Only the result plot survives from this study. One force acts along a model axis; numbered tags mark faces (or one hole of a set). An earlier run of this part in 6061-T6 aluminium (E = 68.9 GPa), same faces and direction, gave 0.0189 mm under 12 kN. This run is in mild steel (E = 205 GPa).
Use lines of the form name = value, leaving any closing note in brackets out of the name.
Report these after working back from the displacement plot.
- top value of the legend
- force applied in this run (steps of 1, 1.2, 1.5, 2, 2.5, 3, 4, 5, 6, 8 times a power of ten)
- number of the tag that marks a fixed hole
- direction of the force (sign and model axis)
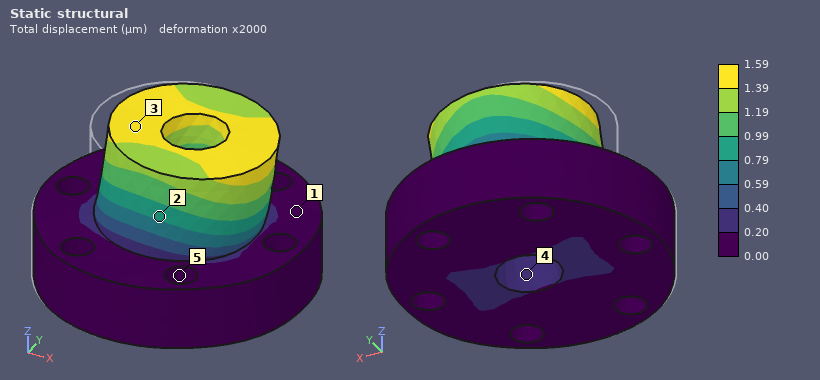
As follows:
top value of the legend = 1.59 µm
force applied in this run = 3 kN
number of the tag that marks a fixed hole = 5
direction of the force = +X
